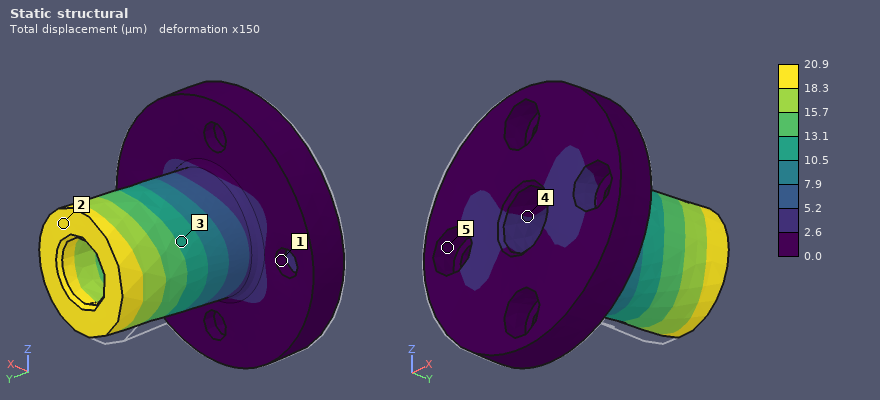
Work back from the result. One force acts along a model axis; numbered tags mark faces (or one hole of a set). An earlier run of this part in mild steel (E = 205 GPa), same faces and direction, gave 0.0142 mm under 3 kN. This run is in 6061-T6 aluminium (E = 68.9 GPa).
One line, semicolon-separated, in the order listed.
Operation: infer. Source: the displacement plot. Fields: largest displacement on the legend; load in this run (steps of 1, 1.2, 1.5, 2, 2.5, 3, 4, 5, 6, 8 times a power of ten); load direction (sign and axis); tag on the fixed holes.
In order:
20.9 µm; 1.5 kN; +X; 1
